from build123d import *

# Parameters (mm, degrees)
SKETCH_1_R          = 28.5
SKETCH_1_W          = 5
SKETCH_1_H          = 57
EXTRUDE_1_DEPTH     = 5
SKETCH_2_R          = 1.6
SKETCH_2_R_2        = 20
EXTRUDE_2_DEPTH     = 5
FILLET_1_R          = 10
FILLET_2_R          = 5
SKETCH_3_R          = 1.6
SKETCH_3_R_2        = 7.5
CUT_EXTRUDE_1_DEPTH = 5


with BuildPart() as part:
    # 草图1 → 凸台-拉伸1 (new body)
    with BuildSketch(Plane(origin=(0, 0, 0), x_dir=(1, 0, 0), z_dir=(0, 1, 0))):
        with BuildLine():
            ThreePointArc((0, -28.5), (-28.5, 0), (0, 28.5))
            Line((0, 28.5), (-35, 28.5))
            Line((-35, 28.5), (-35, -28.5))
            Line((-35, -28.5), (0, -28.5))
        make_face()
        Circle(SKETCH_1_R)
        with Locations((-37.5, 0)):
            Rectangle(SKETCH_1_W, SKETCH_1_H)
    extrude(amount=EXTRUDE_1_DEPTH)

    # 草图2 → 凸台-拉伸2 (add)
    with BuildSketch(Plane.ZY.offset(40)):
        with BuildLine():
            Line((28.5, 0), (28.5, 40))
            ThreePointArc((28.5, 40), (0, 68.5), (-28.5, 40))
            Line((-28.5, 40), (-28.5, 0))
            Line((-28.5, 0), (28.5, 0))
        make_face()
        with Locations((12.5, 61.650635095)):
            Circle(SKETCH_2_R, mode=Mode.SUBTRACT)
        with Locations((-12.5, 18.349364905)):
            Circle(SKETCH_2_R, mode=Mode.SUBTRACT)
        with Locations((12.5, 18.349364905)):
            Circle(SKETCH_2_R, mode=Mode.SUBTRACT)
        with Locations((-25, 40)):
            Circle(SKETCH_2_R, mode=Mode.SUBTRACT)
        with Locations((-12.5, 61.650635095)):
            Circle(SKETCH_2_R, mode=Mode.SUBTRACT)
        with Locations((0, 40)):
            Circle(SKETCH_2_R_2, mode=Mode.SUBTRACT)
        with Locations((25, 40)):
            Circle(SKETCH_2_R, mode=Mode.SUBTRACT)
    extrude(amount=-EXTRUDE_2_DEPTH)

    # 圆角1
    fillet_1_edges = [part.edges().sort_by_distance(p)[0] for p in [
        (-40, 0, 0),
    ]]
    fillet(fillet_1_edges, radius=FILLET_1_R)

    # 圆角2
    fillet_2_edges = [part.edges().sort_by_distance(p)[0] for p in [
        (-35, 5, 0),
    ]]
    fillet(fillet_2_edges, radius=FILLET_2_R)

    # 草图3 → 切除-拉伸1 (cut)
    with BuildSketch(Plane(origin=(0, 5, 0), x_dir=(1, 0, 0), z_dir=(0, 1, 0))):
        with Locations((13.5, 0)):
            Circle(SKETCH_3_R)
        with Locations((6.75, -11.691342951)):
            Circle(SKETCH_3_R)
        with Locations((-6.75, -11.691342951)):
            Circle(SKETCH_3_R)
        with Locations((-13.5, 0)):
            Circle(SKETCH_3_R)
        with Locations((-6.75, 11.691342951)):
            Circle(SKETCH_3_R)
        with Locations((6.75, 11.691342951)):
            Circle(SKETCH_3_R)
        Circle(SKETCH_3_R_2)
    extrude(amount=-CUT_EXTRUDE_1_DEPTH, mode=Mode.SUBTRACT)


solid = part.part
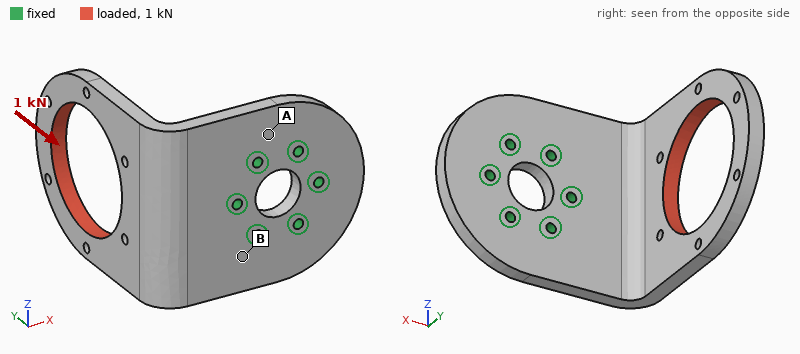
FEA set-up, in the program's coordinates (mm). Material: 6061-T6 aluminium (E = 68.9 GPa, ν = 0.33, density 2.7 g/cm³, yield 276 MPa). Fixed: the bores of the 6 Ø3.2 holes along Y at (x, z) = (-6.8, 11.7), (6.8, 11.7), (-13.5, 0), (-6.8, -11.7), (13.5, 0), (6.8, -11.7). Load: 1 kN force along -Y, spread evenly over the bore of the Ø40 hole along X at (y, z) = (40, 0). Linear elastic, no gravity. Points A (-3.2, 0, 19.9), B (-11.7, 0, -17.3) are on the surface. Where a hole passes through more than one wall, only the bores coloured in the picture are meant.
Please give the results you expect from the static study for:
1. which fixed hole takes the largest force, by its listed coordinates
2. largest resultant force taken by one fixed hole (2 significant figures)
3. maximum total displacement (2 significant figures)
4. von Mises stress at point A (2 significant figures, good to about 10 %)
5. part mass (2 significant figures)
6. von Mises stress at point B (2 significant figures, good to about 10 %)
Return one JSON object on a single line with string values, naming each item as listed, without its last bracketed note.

{"which fixed hole takes the largest force, by its listed coordinates": "(-13.5, 0)", "largest resultant force taken by one fixed hole": "1.3 kN", "maximum total displacement": "0.62 mm", "von Mises stress at point A": "25 MPa", "part mass": "69 g", "von Mises stress at point B": "57 MPa"}
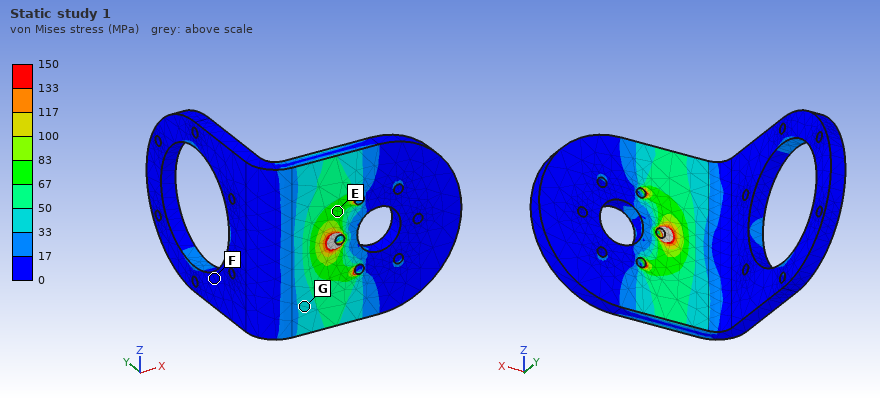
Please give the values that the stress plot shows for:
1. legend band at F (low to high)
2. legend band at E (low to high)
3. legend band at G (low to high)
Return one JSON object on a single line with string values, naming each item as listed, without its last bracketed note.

{"legend band at F": "0 to 17 MPa", "legend band at E": "67 to 83 MPa", "legend band at G": "33 to 50 MPa"}
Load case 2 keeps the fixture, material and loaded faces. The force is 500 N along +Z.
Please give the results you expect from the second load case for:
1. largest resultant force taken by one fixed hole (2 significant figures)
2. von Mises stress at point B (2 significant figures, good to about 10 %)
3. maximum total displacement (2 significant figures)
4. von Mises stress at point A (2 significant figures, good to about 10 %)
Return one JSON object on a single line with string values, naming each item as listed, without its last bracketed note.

{"largest resultant force taken by one fixed hole": "650 N", "von Mises stress at point B": "46 MPa", "maximum total displacement": "0.39 mm", "von Mises stress at point A": "36 MPa"}
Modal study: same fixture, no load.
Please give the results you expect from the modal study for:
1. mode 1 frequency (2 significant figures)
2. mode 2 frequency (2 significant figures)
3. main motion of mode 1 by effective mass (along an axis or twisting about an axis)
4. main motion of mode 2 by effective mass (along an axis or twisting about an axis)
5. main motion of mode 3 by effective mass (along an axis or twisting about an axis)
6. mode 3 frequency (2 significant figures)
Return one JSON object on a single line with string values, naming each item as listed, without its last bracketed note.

{"mode 1 frequency": "830 Hz", "mode 2 frequency": "1400 Hz", "main motion of mode 1 by effective mass": "along X", "main motion of mode 2 by effective mass": "along Z", "main motion of mode 3 by effective mass": "along Y", "mode 3 frequency": "2500 Hz"}
